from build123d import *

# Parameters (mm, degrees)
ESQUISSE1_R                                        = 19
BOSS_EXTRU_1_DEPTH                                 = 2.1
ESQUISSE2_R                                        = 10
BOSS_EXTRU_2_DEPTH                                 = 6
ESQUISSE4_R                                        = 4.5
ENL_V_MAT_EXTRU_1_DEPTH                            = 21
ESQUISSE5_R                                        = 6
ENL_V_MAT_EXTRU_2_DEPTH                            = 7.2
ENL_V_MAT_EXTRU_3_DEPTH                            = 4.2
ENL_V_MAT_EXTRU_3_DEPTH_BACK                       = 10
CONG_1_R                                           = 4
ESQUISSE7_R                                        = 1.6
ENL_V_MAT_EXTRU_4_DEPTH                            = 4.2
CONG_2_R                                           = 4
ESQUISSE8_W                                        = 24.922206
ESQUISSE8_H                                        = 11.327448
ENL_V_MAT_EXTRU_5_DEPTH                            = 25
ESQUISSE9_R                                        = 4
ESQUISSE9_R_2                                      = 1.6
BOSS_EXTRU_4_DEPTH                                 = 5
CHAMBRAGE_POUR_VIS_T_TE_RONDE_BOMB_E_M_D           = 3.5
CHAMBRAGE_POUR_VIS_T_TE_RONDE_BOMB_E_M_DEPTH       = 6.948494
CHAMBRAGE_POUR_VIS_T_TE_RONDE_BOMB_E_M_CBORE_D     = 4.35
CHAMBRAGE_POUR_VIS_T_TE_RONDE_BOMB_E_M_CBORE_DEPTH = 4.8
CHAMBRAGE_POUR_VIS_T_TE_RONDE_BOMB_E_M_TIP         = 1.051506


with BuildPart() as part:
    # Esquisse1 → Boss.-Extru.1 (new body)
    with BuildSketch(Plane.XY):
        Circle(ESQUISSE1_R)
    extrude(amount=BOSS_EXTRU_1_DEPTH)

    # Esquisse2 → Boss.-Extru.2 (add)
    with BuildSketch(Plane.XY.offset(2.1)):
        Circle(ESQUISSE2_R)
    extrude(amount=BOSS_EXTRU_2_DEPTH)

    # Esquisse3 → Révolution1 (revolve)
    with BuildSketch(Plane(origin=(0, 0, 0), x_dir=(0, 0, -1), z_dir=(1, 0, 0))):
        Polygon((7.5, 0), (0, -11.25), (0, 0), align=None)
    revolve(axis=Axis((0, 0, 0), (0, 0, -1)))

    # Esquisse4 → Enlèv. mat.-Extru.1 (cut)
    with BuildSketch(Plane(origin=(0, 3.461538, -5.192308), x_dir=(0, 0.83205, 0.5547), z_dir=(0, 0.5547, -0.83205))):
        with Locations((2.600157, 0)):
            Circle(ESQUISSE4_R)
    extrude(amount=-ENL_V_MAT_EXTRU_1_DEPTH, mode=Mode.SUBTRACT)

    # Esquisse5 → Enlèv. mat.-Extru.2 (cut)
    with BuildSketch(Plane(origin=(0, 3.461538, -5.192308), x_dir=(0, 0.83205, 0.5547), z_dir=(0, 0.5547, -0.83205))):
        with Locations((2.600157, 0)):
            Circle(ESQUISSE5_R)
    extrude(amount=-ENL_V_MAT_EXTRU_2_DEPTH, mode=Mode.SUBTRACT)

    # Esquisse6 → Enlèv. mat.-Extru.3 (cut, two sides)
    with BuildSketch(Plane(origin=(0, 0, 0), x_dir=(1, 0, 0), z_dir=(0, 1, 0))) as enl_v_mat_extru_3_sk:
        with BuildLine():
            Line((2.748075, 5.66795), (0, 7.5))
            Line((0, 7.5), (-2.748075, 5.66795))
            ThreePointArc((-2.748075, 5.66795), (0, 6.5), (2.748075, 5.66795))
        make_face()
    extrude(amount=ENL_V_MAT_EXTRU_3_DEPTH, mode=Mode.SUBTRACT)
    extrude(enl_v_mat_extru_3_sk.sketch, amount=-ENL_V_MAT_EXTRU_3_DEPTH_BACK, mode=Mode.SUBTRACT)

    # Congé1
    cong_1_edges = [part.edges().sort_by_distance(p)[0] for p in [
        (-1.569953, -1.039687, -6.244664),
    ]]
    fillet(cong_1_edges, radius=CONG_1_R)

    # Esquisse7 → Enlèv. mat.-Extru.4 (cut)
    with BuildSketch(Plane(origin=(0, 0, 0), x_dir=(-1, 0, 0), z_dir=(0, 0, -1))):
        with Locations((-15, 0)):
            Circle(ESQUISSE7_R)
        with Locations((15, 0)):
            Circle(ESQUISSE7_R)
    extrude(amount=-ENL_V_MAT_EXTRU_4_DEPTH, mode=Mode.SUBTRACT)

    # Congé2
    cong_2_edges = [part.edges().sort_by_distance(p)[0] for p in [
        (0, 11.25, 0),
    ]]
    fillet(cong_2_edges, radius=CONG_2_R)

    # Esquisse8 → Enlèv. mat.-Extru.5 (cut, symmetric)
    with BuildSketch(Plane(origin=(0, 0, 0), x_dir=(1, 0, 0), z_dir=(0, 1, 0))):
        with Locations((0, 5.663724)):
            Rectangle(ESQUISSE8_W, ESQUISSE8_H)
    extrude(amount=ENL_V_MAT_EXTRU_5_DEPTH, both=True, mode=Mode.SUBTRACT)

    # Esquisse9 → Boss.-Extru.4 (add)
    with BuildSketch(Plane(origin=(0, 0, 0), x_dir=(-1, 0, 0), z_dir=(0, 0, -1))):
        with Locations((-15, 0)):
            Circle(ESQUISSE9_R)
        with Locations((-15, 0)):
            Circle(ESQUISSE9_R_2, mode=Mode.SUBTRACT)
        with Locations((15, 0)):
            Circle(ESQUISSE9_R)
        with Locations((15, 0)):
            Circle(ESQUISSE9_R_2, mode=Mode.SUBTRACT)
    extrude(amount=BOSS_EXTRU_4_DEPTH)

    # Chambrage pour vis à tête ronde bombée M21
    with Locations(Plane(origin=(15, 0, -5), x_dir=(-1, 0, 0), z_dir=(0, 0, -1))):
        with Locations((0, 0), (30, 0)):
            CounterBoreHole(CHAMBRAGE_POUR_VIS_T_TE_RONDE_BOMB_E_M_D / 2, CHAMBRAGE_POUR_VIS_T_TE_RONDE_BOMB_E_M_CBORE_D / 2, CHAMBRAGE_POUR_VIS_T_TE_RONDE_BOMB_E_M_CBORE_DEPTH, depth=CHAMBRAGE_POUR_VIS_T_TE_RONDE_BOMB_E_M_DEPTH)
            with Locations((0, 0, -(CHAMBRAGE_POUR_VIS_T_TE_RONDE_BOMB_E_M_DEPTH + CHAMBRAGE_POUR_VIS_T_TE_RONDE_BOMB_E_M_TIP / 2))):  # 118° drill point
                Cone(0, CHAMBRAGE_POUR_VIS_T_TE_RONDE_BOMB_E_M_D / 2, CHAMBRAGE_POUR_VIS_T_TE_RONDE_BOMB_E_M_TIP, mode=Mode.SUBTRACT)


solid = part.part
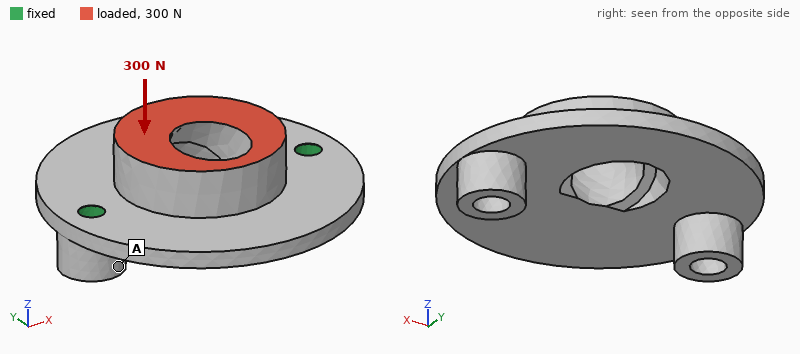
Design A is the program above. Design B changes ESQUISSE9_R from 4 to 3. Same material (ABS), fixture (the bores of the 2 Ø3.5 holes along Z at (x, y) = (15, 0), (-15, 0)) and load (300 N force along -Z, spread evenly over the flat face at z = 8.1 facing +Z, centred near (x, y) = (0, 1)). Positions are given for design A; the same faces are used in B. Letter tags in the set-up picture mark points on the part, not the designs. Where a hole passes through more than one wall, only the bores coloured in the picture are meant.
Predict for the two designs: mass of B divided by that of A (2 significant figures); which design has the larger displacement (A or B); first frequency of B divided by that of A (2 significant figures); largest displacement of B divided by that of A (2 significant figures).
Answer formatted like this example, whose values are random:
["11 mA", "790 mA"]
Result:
["0.94", "B", "0.90", "1.2"]
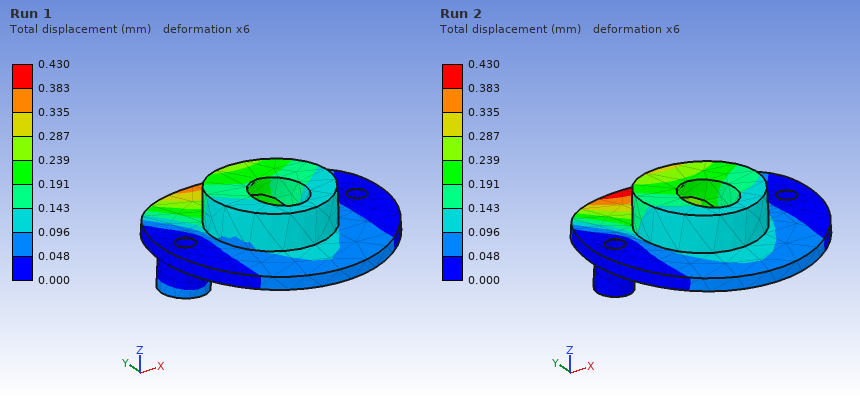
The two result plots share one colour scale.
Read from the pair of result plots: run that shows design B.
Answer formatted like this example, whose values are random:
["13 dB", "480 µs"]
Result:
["Run 2"]
